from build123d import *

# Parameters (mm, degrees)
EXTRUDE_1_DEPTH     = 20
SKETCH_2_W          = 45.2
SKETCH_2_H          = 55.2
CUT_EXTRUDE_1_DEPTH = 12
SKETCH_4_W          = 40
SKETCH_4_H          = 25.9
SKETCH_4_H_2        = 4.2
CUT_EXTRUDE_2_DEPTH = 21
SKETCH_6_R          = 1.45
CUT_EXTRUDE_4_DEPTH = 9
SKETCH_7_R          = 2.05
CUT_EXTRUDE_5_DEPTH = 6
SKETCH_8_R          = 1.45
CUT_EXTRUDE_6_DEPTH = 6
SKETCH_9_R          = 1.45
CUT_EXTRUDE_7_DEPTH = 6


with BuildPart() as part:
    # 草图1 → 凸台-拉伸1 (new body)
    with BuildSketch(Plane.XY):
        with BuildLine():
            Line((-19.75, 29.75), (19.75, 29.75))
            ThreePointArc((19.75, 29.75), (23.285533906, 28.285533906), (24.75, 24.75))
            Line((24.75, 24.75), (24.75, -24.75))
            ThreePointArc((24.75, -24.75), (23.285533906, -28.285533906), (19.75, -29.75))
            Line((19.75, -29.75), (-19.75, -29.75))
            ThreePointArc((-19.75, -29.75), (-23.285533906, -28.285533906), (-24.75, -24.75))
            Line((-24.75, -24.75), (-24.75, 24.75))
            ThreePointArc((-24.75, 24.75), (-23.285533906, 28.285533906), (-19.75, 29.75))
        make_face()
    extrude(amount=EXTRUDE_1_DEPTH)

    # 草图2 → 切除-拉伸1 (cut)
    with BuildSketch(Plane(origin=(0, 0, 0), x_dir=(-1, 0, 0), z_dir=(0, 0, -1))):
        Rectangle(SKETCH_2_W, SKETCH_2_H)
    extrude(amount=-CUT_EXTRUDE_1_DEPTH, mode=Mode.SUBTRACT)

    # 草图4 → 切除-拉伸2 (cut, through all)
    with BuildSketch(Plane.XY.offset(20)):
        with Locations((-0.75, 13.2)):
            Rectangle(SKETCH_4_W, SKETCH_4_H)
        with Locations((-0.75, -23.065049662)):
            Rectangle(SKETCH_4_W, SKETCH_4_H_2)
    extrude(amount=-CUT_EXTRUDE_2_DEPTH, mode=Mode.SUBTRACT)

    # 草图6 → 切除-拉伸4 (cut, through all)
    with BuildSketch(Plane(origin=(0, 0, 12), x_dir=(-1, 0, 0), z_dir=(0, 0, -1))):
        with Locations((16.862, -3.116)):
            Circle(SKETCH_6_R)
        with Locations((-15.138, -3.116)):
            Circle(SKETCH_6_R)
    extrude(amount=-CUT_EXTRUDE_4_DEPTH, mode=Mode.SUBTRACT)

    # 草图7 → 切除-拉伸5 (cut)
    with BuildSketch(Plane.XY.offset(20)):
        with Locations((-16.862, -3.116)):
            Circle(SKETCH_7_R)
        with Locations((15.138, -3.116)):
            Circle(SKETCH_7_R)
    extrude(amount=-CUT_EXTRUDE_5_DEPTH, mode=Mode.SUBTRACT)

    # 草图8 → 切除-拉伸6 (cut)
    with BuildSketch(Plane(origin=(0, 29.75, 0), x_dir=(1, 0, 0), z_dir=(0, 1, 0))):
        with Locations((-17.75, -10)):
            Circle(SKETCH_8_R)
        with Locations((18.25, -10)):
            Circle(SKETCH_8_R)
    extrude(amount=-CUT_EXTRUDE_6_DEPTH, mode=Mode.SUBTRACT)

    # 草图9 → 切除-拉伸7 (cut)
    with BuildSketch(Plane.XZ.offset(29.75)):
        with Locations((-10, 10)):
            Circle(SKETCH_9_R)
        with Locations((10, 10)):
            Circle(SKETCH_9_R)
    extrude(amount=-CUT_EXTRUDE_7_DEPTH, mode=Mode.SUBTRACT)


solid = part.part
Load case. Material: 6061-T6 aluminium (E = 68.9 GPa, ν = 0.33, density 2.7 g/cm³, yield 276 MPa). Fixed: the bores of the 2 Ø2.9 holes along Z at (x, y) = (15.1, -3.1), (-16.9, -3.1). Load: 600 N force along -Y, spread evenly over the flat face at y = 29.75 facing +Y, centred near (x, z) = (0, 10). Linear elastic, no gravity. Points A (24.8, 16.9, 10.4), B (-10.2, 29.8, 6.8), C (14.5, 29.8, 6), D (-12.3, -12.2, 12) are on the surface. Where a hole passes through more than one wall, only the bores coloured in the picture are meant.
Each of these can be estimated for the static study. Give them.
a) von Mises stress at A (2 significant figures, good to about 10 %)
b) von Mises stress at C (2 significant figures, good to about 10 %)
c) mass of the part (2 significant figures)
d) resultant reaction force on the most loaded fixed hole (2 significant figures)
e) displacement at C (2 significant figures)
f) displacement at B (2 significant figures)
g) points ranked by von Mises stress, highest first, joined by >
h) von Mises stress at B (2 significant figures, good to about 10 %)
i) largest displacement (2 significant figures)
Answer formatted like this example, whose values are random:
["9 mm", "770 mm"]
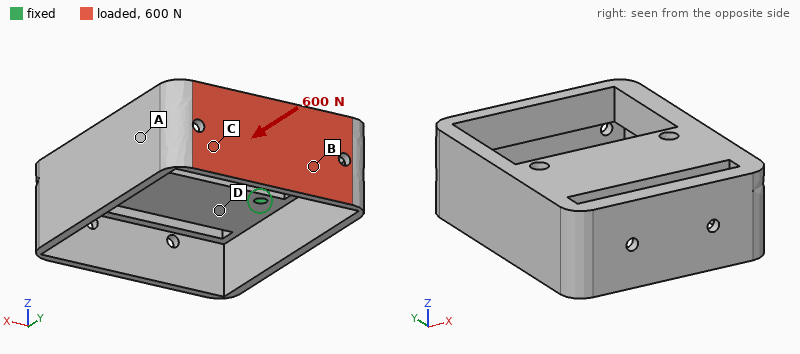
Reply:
["14 MPa", "34 MPa", "50 g", "350 N", "0.10 mm", "0.13 mm", "B > C > A > D", "45 MPa", "0.21 mm"]
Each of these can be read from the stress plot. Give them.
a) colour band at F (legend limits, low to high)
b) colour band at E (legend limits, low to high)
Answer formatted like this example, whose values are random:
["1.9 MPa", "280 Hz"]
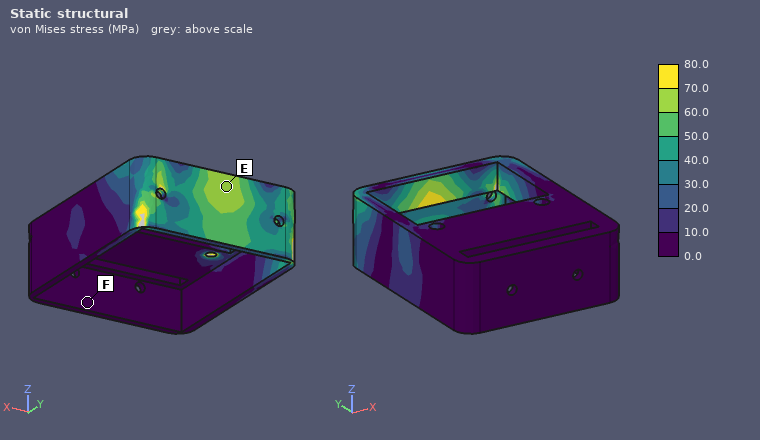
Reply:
["0.0 to 10.0 MPa", "60.0 to 70.0 MPa"]
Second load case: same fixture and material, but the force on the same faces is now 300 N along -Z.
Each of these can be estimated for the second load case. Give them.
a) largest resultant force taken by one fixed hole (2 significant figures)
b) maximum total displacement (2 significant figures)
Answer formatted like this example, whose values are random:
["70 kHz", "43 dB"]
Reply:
["210 N", "0.25 mm"]
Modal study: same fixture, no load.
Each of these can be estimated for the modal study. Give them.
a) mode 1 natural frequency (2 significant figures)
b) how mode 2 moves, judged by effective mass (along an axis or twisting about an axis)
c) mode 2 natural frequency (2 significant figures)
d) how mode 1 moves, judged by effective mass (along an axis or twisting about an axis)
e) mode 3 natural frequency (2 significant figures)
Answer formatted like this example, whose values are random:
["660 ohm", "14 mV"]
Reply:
["1500 Hz", "along X", "2400 Hz", "twisting about X", "4400 Hz"]
